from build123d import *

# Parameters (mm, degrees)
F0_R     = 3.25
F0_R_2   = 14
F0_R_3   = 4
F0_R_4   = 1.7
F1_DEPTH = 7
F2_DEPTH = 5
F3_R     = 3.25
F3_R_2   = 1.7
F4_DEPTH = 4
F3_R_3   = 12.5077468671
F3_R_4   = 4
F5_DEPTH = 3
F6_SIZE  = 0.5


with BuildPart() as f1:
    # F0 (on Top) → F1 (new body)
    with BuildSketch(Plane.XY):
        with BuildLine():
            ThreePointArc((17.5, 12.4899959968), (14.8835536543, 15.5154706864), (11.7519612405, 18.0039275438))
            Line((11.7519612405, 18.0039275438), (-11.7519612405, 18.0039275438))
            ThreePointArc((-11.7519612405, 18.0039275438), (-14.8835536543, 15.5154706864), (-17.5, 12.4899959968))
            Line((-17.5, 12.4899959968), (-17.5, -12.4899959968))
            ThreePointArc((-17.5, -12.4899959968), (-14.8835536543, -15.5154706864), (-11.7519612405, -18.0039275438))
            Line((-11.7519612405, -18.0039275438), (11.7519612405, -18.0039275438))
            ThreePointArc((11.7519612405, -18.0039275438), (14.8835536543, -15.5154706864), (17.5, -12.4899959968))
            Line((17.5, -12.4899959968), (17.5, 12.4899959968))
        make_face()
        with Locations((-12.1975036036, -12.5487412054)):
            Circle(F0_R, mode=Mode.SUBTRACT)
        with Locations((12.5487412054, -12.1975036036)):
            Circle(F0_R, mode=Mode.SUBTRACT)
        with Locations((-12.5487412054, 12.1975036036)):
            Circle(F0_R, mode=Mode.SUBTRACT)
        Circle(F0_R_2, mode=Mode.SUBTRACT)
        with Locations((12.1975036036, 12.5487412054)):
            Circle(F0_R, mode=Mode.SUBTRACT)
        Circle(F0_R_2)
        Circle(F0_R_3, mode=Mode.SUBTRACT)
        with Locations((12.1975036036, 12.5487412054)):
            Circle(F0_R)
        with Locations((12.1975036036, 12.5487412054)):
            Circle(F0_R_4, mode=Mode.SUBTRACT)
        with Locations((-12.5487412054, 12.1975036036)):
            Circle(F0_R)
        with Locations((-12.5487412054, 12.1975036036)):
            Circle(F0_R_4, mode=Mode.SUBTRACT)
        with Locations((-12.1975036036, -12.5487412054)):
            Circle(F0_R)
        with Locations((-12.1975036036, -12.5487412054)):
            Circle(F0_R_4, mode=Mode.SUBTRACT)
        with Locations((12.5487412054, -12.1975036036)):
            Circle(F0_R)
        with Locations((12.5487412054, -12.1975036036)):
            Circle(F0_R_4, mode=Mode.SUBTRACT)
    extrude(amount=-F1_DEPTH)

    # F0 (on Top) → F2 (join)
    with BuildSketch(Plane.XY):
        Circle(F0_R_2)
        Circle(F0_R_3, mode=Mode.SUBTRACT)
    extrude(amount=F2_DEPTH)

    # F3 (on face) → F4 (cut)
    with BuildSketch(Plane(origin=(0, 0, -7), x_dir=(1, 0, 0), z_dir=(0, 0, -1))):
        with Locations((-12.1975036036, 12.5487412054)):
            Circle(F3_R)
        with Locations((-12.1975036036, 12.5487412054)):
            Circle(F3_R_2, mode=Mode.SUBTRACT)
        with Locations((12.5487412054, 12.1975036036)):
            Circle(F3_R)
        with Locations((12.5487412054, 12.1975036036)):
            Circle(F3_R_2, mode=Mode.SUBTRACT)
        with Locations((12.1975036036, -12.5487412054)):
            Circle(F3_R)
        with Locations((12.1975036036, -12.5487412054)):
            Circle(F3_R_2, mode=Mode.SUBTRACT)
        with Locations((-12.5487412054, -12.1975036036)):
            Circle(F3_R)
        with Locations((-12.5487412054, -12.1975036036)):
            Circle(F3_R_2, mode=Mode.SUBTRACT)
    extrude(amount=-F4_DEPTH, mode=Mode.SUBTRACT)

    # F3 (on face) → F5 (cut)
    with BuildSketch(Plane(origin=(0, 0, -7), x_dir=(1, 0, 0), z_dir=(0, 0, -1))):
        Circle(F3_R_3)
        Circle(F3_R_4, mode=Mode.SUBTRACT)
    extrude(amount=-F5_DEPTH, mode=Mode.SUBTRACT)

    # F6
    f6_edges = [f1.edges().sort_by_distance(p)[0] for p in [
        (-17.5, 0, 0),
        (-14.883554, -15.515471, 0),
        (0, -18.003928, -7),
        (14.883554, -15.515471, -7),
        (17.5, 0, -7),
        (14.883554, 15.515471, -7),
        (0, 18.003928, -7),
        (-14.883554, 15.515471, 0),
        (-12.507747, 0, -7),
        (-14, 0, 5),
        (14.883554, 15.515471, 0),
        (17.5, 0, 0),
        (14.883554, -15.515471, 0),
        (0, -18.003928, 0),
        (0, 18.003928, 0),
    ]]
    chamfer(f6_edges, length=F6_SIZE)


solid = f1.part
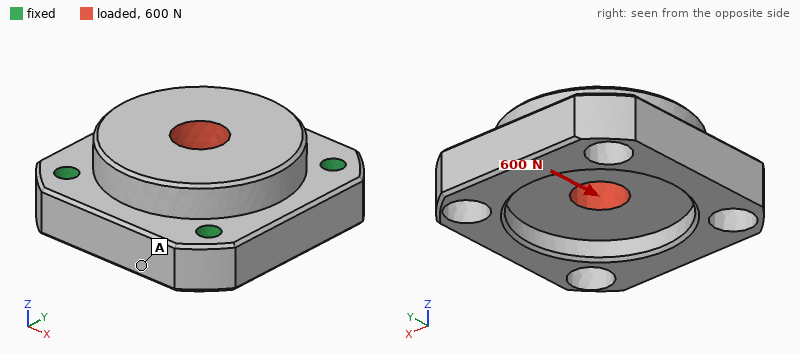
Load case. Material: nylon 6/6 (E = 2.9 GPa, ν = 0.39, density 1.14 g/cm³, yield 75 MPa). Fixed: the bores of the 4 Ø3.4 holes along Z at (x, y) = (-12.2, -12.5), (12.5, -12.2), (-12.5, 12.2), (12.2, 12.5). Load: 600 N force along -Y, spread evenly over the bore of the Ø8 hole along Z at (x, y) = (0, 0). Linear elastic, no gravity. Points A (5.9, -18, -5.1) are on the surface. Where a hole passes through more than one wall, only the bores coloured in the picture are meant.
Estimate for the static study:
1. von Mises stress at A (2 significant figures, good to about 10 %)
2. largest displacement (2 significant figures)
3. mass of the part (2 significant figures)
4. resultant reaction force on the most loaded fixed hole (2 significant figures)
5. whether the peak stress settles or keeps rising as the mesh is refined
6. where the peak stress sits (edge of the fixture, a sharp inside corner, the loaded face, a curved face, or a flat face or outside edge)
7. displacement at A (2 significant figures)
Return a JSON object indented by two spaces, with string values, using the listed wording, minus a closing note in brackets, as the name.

{
  "von Mises stress at A": "1.7 MPa",
  "largest displacement": "25 µm",
  "mass of the part": "10 g",
  "resultant reaction force on the most loaded fixed hole": "160 N",
  "whether the peak stress settles or keeps rising as the mesh is refined": "keeps rising",
  "where the peak stress sits": "edge of the fixture",
  "displacement at A": "12 µm"
}
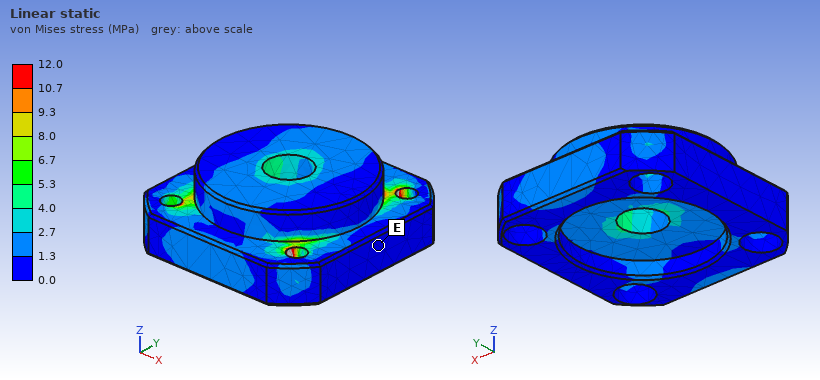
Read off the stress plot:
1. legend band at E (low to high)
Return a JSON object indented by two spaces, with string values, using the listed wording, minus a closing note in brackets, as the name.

{
  "legend band at E": "0.0 to 1.3 MPa"
}
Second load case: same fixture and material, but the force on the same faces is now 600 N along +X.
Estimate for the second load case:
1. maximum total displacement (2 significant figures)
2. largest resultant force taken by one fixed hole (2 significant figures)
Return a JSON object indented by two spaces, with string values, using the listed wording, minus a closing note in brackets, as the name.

{
  "maximum total displacement": "25 µm",
  "largest resultant force taken by one fixed hole": "160 N"
}
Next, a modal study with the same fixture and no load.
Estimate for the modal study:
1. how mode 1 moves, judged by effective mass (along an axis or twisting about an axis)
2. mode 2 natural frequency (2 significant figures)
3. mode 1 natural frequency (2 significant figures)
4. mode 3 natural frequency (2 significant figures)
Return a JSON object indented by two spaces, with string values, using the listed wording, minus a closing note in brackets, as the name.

{
  "how mode 1 moves, judged by effective mass": "along Z",
  "mode 2 natural frequency": "9800 Hz",
  "mode 1 natural frequency": "8000 Hz",
  "mode 3 natural frequency": "9900 Hz"
}
